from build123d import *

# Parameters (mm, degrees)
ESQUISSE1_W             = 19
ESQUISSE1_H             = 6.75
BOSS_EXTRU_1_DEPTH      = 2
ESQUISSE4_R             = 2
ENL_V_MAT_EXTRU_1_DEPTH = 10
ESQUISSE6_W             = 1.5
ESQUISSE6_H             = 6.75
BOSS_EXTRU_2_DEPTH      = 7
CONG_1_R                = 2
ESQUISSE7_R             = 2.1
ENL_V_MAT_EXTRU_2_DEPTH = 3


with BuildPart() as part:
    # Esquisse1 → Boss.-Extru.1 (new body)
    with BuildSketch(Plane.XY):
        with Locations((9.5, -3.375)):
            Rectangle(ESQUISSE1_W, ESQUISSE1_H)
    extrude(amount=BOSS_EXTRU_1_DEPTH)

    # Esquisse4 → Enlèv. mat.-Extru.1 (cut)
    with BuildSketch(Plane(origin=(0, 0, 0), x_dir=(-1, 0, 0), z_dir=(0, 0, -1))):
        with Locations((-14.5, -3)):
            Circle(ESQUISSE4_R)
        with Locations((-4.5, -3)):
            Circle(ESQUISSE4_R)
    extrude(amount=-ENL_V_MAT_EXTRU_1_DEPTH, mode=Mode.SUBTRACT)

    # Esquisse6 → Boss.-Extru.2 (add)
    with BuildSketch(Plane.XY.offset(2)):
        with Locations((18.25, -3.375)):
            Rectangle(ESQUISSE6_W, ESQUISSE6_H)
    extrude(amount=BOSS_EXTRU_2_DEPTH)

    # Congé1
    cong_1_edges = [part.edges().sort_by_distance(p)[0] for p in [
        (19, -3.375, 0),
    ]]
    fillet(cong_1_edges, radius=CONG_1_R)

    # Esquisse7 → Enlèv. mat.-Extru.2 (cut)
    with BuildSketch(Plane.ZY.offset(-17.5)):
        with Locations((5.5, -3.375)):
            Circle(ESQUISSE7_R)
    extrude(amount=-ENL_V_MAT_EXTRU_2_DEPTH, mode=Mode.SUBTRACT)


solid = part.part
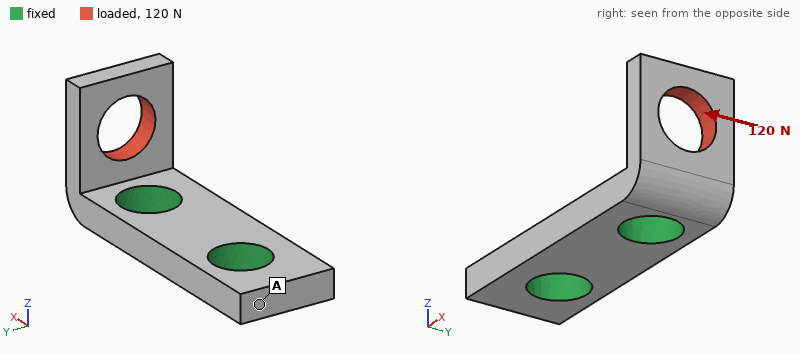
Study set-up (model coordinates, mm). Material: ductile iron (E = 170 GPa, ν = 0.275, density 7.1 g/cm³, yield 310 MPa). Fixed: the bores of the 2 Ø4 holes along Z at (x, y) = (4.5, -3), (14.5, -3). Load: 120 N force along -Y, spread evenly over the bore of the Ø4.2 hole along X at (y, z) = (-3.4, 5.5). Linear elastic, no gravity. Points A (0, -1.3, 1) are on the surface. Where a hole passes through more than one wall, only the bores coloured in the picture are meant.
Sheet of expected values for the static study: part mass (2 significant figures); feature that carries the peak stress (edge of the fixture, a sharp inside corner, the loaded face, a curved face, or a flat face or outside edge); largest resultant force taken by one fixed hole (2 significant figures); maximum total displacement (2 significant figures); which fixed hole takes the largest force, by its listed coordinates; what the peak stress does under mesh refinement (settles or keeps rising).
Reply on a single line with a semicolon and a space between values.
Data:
1.8 g; edge of the fixture; 120 N; 13 µm; (14.5, -3); keeps rising
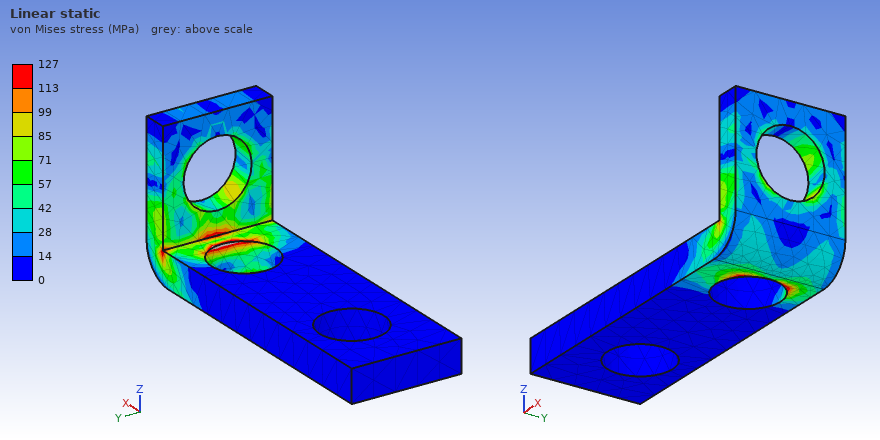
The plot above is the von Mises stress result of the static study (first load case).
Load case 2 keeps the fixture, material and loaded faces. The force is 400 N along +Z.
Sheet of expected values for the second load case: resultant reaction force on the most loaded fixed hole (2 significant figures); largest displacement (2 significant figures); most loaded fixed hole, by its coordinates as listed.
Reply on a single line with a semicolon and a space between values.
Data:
400 N; 16 µm; (14.5, -3)
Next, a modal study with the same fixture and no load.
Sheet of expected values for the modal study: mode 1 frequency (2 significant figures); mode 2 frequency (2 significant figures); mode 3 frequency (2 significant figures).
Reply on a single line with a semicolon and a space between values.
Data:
16 kHz; 29 kHz; 37 kHz
